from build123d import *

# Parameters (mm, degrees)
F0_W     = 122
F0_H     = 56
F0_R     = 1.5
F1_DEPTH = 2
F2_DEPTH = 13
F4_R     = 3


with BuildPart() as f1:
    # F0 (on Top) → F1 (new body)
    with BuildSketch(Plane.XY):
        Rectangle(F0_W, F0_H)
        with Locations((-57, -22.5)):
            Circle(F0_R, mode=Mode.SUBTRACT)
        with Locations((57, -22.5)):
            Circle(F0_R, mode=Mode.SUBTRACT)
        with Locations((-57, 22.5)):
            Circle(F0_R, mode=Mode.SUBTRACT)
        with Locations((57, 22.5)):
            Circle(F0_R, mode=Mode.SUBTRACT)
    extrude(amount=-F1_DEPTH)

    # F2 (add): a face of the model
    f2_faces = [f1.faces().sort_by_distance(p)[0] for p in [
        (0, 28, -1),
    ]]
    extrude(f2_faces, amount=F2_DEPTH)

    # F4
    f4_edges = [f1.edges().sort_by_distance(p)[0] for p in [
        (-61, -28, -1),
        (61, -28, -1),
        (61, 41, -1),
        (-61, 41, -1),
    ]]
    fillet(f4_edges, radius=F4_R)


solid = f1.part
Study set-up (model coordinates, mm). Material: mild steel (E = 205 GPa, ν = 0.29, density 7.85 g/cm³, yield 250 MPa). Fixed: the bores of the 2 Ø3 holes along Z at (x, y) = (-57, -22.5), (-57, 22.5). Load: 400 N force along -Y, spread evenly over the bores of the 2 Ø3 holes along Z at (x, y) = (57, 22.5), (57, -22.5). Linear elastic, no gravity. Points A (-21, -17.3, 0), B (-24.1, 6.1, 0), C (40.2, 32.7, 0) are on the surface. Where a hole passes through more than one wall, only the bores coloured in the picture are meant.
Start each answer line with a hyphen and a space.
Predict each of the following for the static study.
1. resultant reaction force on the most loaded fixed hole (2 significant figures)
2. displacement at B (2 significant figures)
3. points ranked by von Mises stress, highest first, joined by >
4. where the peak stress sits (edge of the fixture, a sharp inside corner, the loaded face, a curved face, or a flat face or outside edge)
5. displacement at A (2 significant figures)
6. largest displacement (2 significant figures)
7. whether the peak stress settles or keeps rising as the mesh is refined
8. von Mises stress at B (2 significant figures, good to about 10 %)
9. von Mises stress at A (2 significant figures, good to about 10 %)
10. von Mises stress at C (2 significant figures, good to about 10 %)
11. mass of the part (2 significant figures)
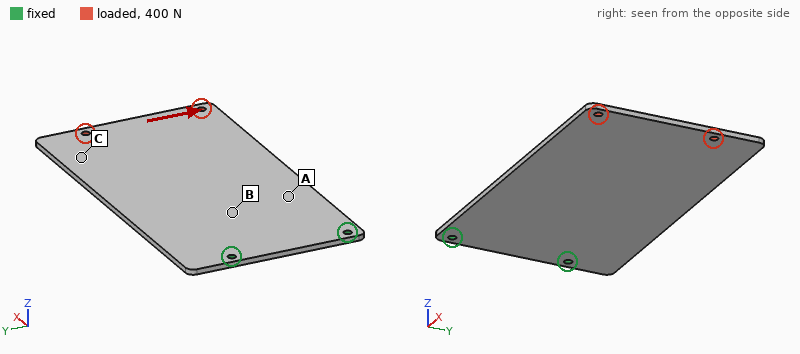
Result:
- 1.0 kN
- 6.3 µm
- A > B > C
- edge of the fixture
- 8.2 µm
- 36 µm
- keeps rising
- 9.3 MPa
- 16 MPa
- 4.6 MPa
- 130 g
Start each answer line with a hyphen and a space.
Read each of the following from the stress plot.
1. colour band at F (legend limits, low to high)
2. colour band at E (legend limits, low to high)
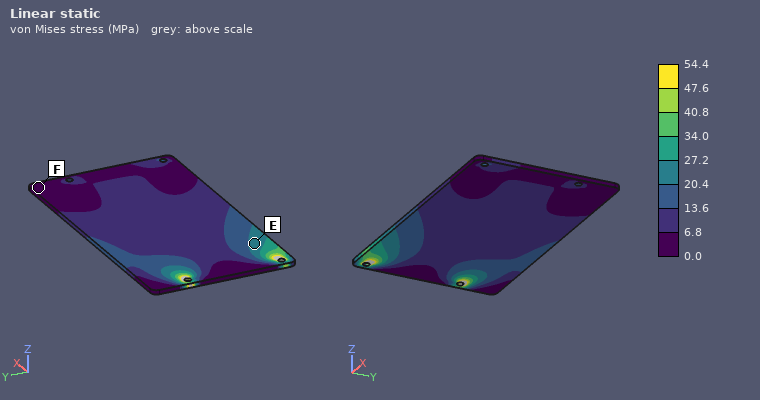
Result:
- 0.0 to 6.8 MPa
- 20.4 to 27.2 MPa
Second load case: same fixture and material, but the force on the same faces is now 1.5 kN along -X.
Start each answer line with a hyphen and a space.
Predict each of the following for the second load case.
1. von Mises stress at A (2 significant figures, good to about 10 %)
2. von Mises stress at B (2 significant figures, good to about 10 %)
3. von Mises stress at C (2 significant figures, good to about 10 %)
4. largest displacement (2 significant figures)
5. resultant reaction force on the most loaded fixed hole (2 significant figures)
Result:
- 15 MPa
- 9.5 MPa
- 9.0 MPa
- 14 µm
- 770 N
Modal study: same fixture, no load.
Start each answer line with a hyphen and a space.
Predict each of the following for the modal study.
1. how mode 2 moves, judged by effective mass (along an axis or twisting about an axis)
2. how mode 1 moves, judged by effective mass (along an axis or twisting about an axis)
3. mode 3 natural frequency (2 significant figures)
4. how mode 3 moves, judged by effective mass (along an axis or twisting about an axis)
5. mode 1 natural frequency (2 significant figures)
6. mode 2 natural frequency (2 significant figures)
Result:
- twisting about X
- along Z
- 710 Hz
- along Z
- 110 Hz
- 440 Hz
